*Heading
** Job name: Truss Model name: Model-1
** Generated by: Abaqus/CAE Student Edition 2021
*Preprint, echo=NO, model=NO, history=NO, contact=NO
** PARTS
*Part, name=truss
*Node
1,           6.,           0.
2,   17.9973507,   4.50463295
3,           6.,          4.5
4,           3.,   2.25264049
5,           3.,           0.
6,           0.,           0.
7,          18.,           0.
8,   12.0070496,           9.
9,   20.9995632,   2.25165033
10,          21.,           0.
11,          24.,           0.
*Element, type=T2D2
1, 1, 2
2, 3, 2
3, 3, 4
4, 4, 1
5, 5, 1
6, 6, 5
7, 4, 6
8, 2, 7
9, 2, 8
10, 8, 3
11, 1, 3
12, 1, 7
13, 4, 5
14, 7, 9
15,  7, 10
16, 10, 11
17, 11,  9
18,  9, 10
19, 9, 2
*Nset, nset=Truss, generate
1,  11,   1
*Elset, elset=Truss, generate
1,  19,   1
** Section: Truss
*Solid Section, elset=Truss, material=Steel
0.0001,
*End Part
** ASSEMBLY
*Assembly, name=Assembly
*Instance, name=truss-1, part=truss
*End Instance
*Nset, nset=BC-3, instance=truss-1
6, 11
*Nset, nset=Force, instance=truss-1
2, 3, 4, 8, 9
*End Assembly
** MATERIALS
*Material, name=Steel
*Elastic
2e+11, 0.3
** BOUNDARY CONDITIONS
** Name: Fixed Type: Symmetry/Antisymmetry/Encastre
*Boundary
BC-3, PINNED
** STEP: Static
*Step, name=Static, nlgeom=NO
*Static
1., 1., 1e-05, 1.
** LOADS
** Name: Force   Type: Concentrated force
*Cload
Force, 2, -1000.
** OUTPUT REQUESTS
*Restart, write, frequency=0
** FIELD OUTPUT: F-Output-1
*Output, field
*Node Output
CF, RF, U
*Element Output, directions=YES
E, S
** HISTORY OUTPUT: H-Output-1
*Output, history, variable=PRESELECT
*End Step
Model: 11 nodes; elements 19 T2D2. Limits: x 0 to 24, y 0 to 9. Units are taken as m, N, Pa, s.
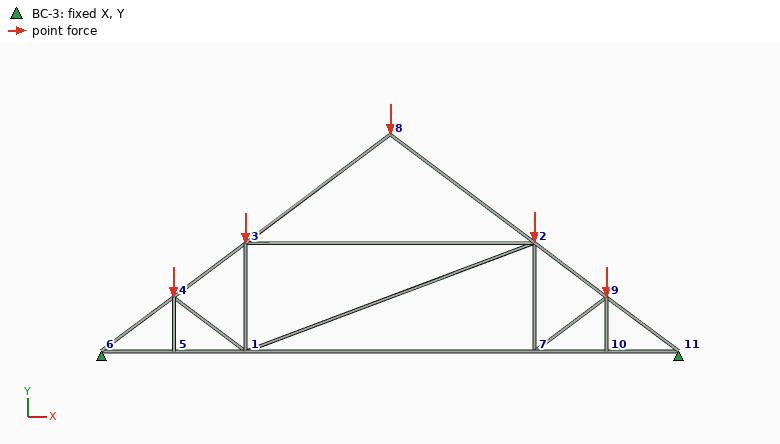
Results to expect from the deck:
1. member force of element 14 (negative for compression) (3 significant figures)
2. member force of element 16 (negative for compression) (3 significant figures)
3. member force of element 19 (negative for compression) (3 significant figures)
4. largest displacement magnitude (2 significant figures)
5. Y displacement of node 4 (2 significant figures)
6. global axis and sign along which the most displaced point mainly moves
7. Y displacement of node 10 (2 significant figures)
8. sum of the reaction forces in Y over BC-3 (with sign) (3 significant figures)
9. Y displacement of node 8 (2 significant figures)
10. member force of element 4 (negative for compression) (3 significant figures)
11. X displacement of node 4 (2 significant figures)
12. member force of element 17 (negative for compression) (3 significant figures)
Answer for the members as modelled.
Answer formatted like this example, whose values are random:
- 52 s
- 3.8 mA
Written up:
- -833 N
- 334 N
- -3330 N
- 0.0037 m
- -0.0027 m
- -Y
- -0.0023 m
- 5000 N
- -0.0029 m
- -829 N
- 0.0010 m
- -4170 N
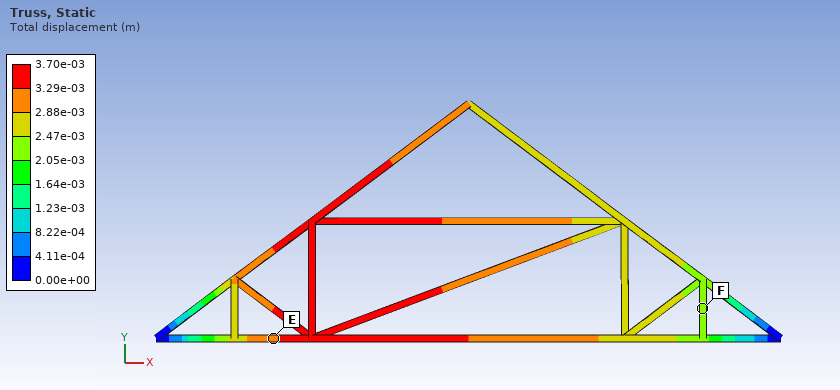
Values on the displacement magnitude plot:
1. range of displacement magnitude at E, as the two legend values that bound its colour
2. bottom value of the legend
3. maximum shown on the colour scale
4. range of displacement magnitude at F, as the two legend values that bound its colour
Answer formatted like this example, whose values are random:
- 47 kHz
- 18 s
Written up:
- 2.88e-03 to 3.29e-03 m
- 0.00e+00 m
- 3.70e-03 m
- 2.05e-03 to 2.47e-03 m
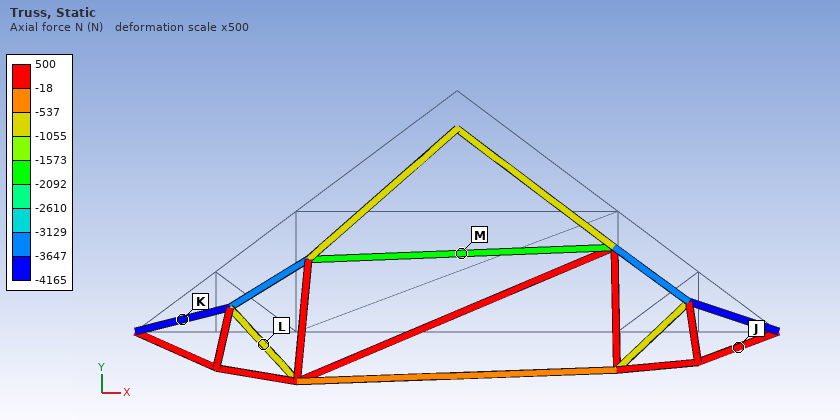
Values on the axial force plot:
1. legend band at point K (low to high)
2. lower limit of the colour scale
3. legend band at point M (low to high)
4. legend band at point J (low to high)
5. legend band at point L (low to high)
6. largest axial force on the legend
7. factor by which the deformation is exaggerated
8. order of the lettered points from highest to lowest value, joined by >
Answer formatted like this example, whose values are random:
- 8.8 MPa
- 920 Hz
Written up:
- -4165 to -3647 N
- -4165 N
- -2092 to -1573 N
- -18 to 500 N
- -1055 to -537 N
- 500 N
- 500
- J > L > M > K
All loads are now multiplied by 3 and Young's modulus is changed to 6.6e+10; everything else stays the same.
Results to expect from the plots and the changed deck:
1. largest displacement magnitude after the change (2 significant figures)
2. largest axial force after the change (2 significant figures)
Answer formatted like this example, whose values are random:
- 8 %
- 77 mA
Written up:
- 0.034 m
- 1500 N
